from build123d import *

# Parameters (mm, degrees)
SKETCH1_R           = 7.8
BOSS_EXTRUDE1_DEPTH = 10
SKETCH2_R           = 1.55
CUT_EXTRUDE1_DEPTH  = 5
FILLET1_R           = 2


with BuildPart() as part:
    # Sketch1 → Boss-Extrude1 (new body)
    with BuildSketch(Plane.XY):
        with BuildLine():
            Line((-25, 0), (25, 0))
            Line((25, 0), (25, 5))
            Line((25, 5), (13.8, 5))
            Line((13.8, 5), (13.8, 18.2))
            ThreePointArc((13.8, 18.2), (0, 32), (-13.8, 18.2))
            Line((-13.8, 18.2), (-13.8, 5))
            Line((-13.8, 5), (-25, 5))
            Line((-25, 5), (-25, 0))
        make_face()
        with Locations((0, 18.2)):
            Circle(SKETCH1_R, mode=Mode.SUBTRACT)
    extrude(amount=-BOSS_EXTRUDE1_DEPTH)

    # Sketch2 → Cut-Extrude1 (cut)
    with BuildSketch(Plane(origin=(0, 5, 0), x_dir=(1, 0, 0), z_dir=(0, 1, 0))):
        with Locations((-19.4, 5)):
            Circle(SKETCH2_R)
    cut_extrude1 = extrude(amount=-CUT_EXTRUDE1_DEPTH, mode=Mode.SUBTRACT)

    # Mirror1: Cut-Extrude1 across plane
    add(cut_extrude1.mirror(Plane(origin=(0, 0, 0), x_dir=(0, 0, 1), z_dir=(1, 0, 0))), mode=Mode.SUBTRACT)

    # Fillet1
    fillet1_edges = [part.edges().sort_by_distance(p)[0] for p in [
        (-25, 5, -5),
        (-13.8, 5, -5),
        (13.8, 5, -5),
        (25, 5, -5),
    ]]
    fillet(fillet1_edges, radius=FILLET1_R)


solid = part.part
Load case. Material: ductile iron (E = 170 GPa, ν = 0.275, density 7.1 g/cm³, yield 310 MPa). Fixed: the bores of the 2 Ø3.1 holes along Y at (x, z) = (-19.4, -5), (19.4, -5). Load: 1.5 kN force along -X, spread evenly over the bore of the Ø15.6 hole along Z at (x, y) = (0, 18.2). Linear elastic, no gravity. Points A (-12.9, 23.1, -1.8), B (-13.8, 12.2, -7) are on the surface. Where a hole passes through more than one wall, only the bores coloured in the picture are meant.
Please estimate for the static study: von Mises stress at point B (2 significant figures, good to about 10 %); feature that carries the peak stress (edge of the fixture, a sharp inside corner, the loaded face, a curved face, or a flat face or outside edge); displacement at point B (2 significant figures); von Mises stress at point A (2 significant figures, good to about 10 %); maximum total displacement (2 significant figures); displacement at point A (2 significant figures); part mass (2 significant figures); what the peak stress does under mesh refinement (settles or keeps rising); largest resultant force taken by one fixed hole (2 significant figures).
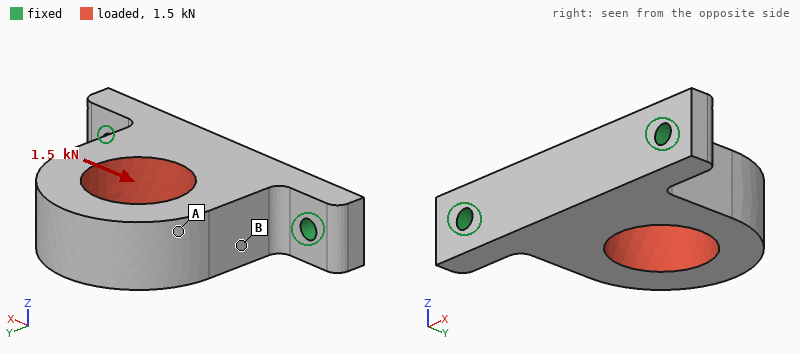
26 MPa
edge of the fixture
4.6 µm
11 MPa
12 µm
10.0 µm
51 g
keeps rising
1.0 kN
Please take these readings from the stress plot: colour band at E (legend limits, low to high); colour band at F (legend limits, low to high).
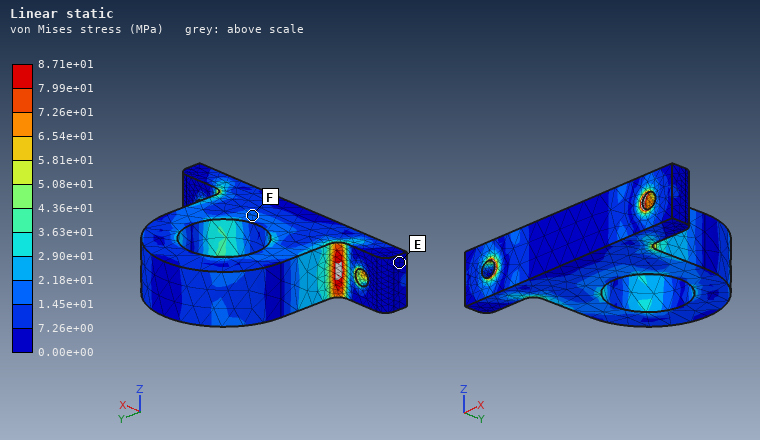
0.00e+00 to 7.26e+00 MPa
1.45e+01 to 2.18e+01 MPa
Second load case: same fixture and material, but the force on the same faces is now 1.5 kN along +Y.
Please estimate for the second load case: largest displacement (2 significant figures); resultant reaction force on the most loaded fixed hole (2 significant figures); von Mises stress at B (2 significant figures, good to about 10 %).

4.6 µm
840 N
14 MPa
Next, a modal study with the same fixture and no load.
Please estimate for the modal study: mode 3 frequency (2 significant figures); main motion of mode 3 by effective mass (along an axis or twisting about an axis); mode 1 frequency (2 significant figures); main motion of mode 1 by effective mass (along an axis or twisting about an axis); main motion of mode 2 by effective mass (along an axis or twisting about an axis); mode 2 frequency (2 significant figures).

15 kHz
along Y
3900 Hz
along Z
along X
12 kHz
